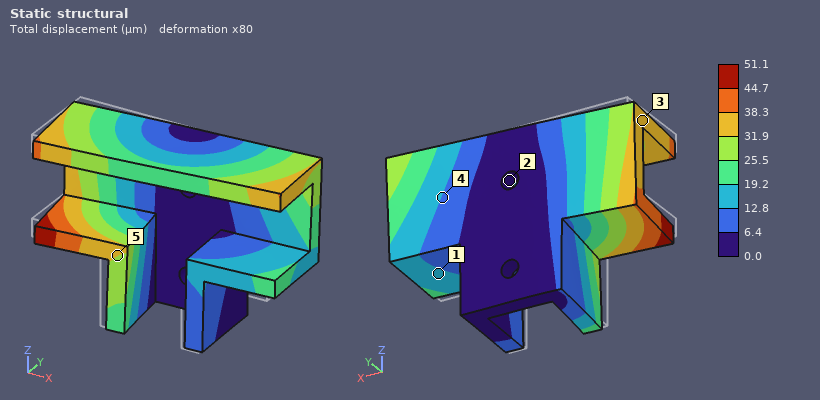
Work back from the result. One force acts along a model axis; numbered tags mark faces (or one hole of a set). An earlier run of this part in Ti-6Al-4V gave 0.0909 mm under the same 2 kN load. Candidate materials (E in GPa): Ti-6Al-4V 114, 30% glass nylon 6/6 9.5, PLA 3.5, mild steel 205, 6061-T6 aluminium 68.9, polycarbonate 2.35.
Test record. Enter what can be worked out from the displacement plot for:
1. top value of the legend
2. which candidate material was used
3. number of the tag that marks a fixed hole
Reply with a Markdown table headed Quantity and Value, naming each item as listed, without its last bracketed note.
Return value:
| Quantity | Value |
|---|---|
| top value of the legend | 51.1 µm |
| which candidate material was used | mild steel |
| number of the tag that marks a fixed hole | 2 |
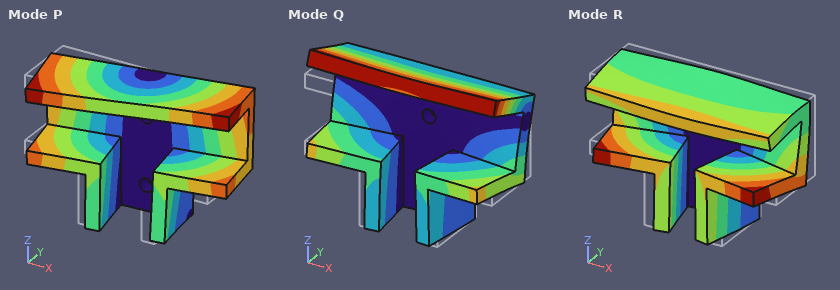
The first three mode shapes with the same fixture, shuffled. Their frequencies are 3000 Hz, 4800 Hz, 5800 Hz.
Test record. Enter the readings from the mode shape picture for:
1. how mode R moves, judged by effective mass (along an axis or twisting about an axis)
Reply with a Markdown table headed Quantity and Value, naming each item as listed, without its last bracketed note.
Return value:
| Quantity | Value |
|---|---|
| how mode R moves, judged by effective mass | along Y |
